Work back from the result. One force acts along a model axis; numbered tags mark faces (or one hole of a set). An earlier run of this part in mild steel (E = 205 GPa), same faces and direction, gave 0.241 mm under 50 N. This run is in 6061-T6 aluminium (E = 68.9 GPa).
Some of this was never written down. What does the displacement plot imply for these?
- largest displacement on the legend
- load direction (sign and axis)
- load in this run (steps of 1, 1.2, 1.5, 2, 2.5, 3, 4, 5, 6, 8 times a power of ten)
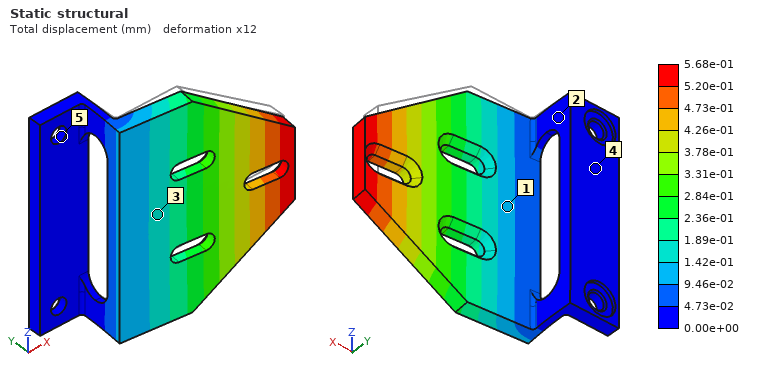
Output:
5.68e-01 mm
-Y
40 N
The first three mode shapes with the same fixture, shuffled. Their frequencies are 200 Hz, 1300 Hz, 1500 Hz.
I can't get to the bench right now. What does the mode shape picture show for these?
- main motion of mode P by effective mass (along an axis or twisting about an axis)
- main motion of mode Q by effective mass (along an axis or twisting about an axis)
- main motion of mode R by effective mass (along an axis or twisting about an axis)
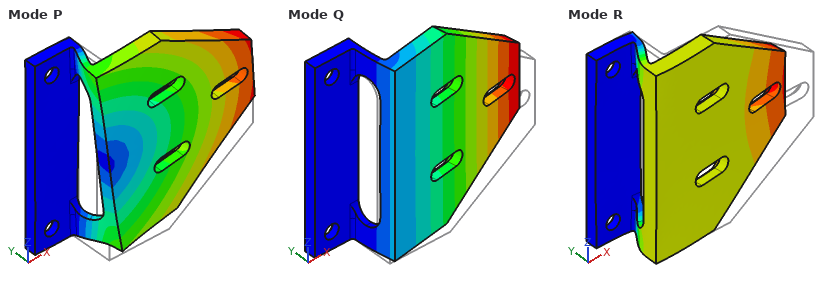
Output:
along Z
along Y
along X
